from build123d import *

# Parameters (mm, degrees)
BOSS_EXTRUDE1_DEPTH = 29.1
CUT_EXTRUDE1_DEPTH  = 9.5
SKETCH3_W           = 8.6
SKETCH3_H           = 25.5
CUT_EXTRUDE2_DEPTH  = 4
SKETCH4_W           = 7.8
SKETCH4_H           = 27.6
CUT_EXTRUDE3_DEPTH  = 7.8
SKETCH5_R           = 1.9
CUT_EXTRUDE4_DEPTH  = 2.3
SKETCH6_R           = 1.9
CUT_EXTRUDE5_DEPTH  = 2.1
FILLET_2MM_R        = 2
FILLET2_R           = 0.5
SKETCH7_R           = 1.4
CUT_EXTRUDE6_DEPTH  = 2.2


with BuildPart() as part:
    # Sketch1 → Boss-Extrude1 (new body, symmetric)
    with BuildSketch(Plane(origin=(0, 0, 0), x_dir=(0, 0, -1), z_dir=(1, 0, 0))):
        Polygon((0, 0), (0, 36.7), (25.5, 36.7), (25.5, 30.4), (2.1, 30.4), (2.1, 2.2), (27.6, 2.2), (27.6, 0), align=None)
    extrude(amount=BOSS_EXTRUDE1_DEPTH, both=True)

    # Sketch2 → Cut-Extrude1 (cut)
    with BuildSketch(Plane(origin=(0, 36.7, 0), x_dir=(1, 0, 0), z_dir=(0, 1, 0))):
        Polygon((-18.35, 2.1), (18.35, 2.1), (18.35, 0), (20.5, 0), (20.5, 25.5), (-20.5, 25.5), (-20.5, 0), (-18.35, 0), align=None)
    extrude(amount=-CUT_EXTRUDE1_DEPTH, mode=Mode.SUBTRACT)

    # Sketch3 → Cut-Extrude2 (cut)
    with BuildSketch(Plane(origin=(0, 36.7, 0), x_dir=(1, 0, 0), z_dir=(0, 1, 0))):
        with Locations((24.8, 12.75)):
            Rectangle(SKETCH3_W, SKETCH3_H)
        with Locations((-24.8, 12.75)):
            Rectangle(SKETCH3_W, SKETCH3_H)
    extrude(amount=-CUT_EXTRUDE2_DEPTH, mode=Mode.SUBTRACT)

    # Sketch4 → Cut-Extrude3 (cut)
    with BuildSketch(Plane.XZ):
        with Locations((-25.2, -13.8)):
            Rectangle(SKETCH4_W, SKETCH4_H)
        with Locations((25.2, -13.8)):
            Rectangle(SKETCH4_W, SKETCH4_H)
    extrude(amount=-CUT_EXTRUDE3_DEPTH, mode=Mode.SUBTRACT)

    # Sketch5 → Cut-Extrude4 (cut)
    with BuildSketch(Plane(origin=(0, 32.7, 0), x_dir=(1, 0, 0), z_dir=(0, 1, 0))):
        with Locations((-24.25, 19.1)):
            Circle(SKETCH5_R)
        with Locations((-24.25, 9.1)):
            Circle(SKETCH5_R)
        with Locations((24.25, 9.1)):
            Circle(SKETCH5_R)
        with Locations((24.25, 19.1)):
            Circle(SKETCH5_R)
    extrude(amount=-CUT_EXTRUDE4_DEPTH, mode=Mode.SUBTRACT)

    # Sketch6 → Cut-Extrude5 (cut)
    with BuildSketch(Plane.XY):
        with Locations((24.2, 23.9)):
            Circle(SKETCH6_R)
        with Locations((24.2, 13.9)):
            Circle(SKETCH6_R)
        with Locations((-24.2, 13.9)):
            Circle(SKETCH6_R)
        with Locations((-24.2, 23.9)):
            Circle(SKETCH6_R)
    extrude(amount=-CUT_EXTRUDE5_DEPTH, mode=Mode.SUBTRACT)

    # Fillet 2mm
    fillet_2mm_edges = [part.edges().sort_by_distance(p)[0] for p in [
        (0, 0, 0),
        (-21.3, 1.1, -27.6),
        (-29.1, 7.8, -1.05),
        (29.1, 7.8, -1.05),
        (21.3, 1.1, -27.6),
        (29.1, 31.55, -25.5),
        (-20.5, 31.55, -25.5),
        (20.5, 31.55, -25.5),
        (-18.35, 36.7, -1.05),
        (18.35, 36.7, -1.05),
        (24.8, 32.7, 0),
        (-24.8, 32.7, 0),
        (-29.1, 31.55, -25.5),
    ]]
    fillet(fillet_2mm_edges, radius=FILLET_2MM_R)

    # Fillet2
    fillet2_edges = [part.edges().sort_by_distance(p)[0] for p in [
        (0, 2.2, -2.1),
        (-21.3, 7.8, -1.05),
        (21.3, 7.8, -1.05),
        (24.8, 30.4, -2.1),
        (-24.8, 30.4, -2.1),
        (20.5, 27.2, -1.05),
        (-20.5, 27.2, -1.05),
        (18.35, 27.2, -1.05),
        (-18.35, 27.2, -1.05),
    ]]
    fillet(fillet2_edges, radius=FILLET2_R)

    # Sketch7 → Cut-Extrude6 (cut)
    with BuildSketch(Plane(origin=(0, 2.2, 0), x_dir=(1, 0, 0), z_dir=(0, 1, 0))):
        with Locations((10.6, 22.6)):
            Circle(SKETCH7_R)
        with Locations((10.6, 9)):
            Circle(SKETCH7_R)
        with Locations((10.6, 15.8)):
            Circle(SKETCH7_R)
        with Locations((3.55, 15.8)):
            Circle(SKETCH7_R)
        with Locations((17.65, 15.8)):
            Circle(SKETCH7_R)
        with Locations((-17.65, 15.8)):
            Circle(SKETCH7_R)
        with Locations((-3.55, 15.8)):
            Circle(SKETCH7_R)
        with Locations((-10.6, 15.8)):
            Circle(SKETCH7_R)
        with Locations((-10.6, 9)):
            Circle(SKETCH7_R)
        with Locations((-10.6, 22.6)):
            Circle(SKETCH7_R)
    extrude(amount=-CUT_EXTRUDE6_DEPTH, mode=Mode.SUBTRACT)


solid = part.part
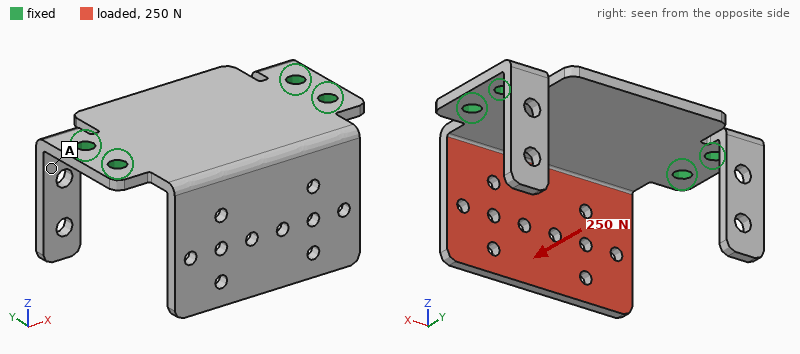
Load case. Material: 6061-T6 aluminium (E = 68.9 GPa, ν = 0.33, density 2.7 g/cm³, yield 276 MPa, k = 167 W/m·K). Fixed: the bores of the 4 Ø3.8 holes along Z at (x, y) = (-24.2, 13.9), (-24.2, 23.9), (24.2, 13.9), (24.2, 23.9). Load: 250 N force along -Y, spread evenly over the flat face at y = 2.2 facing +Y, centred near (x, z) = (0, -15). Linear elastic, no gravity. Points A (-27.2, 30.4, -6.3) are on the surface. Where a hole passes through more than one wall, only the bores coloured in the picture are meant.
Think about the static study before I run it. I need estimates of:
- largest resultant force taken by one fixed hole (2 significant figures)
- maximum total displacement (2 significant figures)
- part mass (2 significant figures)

110 N
0.78 mm
19 g
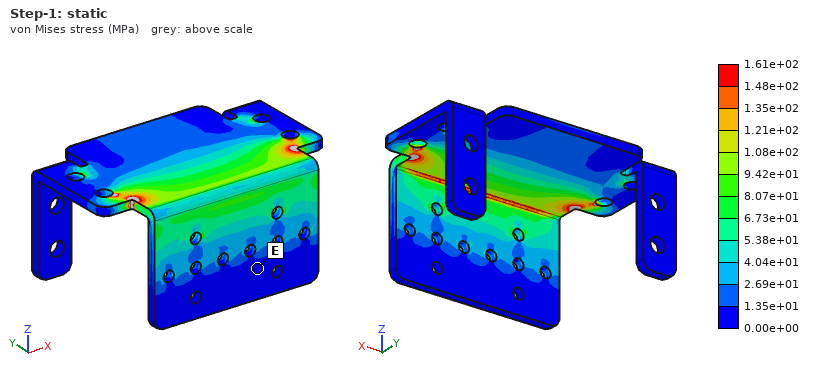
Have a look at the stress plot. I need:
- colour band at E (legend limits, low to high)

0.00e+00 to 1.35e+01 MPa
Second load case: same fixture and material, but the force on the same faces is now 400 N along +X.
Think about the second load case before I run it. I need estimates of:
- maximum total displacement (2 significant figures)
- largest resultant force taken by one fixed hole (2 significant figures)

0.20 mm
230 N
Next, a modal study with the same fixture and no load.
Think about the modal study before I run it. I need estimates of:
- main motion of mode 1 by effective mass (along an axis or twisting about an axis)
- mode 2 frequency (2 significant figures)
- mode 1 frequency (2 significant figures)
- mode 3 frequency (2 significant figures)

along Y
2200 Hz
1300 Hz
2200 Hz
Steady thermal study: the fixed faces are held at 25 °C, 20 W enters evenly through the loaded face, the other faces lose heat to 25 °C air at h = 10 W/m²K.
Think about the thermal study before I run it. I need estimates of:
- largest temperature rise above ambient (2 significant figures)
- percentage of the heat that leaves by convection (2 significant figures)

44 K
4.8 %
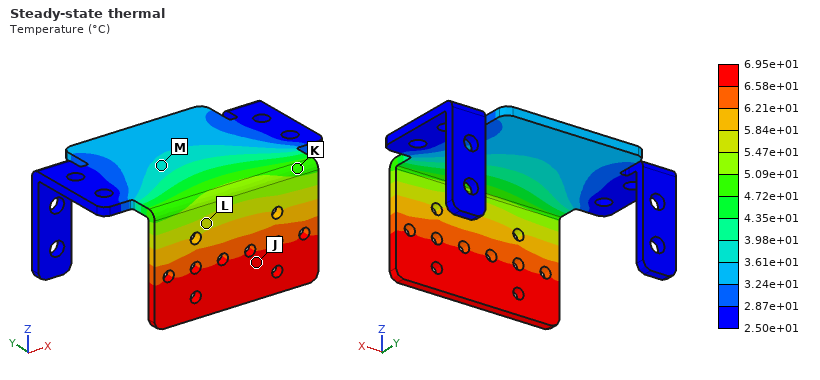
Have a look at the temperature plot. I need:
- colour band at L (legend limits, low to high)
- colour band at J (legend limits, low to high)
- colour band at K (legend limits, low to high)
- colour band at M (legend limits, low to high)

5.47e+01 to 5.84e+01 °C
6.58e+01 to 6.95e+01 °C
4.72e+01 to 5.09e+01 °C
3.61e+01 to 3.98e+01 °C
